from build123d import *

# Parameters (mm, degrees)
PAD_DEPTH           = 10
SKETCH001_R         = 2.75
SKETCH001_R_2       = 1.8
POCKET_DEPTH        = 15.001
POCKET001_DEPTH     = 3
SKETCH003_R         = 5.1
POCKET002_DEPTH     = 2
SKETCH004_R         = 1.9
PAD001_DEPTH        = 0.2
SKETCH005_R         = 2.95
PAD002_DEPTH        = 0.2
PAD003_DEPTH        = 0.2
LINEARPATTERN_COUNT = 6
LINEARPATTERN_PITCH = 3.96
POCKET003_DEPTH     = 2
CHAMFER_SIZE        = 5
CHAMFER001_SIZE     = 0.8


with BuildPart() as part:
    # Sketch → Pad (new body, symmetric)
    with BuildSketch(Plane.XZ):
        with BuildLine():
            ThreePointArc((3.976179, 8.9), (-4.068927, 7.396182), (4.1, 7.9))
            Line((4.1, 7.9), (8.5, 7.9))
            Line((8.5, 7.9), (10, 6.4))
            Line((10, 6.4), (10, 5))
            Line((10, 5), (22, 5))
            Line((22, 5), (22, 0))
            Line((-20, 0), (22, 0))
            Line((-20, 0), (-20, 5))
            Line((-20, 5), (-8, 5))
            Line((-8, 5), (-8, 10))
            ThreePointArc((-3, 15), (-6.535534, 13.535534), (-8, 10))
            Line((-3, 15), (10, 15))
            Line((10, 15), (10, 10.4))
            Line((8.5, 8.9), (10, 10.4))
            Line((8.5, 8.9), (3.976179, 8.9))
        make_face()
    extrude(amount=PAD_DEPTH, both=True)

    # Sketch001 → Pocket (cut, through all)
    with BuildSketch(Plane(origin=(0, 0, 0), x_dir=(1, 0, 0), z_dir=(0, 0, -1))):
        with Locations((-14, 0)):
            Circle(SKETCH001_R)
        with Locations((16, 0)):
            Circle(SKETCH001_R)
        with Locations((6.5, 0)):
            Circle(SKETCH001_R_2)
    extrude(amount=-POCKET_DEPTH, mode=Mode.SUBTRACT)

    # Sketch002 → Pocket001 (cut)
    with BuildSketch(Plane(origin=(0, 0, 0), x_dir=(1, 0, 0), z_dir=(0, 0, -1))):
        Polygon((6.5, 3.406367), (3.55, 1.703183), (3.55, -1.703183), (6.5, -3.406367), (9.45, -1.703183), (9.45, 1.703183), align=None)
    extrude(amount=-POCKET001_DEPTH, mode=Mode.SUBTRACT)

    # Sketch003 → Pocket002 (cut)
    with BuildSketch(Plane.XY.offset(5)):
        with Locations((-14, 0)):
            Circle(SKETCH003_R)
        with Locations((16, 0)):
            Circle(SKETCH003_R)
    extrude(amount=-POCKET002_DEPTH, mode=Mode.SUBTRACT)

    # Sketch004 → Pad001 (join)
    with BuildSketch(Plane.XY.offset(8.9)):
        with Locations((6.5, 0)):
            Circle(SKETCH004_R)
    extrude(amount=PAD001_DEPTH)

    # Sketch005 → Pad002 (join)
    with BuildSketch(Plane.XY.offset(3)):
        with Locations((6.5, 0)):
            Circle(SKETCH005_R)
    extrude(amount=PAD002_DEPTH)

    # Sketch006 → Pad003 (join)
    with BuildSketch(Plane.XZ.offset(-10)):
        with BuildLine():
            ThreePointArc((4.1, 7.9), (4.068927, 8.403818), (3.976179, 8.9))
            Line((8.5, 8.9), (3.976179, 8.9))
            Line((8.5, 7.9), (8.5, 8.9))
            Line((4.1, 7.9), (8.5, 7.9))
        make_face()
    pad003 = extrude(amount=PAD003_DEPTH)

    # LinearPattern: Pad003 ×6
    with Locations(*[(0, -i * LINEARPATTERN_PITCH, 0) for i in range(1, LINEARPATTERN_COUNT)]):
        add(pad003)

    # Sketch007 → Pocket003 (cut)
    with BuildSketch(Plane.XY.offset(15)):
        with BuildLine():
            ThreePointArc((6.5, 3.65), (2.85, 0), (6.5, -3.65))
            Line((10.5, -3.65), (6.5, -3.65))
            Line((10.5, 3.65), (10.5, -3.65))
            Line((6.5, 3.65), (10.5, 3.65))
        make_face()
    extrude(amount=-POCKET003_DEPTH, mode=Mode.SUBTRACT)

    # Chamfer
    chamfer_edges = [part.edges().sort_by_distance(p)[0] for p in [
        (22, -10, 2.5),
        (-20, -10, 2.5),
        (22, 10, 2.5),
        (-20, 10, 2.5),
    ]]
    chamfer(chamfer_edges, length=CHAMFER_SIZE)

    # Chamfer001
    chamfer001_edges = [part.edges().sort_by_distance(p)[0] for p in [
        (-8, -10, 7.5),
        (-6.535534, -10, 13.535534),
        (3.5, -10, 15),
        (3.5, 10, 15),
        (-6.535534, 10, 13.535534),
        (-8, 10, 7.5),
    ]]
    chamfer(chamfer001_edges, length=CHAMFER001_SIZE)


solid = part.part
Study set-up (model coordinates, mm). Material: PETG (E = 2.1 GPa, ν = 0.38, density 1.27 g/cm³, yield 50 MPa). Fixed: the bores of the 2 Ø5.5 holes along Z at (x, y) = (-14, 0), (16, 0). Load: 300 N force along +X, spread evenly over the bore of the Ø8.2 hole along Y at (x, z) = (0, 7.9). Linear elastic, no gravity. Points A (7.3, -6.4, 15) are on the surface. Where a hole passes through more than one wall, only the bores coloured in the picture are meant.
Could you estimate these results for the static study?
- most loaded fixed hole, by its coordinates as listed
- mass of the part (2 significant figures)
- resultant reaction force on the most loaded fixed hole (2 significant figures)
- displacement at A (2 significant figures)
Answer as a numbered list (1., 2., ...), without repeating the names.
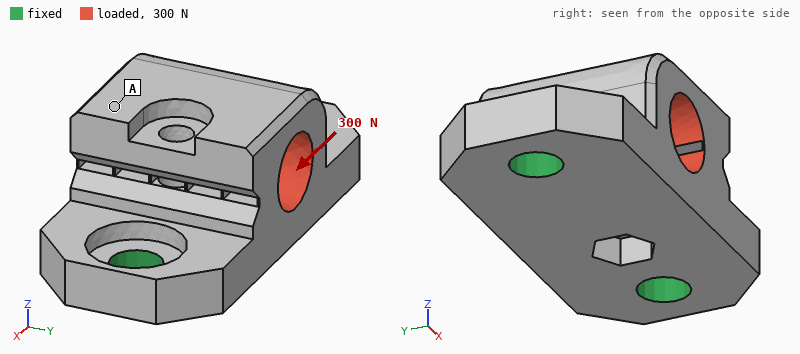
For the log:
1. (-14, 0)
2. 6.9 g
3. 180 N
4. 63 µm
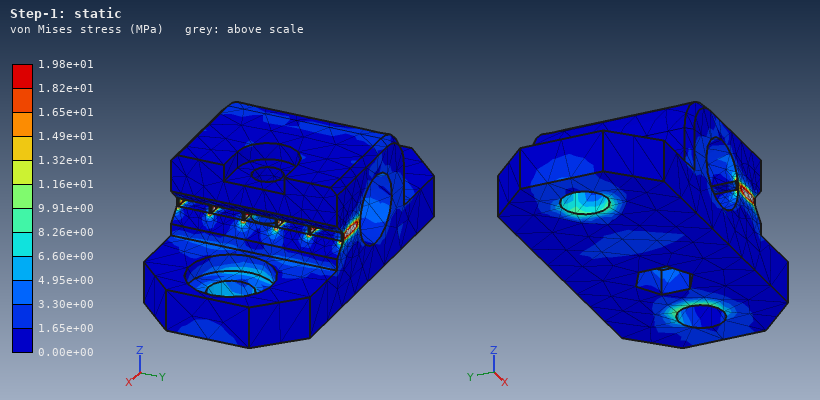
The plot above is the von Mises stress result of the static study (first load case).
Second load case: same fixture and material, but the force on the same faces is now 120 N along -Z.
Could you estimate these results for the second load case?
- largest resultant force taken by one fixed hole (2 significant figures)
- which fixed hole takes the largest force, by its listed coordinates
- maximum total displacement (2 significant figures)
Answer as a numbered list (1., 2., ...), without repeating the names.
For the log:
1. 74 N
2. (-14, 0)
3. 39 µm
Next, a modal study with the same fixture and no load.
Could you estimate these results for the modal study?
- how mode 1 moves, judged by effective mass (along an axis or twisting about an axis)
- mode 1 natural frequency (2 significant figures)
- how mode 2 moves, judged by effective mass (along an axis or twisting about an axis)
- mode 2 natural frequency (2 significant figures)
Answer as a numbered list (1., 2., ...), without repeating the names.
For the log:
1. along Y
2. 2300 Hz
3. along Z
4. 4400 Hz
